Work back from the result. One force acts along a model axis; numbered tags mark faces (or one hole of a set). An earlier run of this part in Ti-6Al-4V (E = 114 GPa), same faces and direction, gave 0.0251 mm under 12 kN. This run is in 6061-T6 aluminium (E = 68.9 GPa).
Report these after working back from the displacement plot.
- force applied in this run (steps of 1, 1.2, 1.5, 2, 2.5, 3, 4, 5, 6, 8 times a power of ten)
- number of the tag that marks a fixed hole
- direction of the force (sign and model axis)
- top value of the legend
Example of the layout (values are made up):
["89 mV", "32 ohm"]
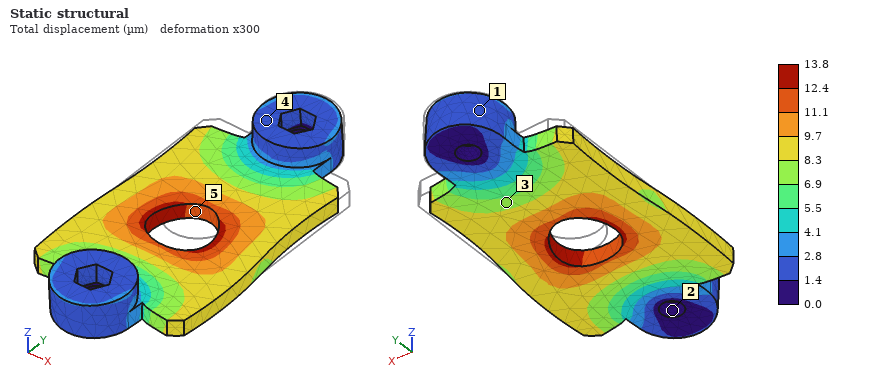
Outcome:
["4 kN", "2", "-Y", "13.8 µm"]
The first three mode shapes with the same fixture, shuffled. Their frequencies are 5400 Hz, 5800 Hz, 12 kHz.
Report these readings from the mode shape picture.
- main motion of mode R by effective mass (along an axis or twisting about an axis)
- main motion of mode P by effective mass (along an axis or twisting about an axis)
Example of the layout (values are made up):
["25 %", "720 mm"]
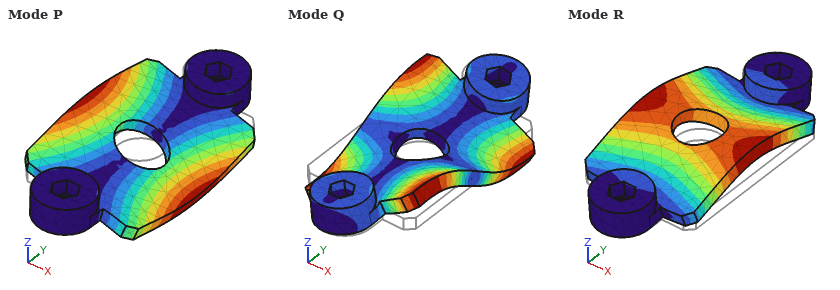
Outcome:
["along Z", "twisting about Y"]
